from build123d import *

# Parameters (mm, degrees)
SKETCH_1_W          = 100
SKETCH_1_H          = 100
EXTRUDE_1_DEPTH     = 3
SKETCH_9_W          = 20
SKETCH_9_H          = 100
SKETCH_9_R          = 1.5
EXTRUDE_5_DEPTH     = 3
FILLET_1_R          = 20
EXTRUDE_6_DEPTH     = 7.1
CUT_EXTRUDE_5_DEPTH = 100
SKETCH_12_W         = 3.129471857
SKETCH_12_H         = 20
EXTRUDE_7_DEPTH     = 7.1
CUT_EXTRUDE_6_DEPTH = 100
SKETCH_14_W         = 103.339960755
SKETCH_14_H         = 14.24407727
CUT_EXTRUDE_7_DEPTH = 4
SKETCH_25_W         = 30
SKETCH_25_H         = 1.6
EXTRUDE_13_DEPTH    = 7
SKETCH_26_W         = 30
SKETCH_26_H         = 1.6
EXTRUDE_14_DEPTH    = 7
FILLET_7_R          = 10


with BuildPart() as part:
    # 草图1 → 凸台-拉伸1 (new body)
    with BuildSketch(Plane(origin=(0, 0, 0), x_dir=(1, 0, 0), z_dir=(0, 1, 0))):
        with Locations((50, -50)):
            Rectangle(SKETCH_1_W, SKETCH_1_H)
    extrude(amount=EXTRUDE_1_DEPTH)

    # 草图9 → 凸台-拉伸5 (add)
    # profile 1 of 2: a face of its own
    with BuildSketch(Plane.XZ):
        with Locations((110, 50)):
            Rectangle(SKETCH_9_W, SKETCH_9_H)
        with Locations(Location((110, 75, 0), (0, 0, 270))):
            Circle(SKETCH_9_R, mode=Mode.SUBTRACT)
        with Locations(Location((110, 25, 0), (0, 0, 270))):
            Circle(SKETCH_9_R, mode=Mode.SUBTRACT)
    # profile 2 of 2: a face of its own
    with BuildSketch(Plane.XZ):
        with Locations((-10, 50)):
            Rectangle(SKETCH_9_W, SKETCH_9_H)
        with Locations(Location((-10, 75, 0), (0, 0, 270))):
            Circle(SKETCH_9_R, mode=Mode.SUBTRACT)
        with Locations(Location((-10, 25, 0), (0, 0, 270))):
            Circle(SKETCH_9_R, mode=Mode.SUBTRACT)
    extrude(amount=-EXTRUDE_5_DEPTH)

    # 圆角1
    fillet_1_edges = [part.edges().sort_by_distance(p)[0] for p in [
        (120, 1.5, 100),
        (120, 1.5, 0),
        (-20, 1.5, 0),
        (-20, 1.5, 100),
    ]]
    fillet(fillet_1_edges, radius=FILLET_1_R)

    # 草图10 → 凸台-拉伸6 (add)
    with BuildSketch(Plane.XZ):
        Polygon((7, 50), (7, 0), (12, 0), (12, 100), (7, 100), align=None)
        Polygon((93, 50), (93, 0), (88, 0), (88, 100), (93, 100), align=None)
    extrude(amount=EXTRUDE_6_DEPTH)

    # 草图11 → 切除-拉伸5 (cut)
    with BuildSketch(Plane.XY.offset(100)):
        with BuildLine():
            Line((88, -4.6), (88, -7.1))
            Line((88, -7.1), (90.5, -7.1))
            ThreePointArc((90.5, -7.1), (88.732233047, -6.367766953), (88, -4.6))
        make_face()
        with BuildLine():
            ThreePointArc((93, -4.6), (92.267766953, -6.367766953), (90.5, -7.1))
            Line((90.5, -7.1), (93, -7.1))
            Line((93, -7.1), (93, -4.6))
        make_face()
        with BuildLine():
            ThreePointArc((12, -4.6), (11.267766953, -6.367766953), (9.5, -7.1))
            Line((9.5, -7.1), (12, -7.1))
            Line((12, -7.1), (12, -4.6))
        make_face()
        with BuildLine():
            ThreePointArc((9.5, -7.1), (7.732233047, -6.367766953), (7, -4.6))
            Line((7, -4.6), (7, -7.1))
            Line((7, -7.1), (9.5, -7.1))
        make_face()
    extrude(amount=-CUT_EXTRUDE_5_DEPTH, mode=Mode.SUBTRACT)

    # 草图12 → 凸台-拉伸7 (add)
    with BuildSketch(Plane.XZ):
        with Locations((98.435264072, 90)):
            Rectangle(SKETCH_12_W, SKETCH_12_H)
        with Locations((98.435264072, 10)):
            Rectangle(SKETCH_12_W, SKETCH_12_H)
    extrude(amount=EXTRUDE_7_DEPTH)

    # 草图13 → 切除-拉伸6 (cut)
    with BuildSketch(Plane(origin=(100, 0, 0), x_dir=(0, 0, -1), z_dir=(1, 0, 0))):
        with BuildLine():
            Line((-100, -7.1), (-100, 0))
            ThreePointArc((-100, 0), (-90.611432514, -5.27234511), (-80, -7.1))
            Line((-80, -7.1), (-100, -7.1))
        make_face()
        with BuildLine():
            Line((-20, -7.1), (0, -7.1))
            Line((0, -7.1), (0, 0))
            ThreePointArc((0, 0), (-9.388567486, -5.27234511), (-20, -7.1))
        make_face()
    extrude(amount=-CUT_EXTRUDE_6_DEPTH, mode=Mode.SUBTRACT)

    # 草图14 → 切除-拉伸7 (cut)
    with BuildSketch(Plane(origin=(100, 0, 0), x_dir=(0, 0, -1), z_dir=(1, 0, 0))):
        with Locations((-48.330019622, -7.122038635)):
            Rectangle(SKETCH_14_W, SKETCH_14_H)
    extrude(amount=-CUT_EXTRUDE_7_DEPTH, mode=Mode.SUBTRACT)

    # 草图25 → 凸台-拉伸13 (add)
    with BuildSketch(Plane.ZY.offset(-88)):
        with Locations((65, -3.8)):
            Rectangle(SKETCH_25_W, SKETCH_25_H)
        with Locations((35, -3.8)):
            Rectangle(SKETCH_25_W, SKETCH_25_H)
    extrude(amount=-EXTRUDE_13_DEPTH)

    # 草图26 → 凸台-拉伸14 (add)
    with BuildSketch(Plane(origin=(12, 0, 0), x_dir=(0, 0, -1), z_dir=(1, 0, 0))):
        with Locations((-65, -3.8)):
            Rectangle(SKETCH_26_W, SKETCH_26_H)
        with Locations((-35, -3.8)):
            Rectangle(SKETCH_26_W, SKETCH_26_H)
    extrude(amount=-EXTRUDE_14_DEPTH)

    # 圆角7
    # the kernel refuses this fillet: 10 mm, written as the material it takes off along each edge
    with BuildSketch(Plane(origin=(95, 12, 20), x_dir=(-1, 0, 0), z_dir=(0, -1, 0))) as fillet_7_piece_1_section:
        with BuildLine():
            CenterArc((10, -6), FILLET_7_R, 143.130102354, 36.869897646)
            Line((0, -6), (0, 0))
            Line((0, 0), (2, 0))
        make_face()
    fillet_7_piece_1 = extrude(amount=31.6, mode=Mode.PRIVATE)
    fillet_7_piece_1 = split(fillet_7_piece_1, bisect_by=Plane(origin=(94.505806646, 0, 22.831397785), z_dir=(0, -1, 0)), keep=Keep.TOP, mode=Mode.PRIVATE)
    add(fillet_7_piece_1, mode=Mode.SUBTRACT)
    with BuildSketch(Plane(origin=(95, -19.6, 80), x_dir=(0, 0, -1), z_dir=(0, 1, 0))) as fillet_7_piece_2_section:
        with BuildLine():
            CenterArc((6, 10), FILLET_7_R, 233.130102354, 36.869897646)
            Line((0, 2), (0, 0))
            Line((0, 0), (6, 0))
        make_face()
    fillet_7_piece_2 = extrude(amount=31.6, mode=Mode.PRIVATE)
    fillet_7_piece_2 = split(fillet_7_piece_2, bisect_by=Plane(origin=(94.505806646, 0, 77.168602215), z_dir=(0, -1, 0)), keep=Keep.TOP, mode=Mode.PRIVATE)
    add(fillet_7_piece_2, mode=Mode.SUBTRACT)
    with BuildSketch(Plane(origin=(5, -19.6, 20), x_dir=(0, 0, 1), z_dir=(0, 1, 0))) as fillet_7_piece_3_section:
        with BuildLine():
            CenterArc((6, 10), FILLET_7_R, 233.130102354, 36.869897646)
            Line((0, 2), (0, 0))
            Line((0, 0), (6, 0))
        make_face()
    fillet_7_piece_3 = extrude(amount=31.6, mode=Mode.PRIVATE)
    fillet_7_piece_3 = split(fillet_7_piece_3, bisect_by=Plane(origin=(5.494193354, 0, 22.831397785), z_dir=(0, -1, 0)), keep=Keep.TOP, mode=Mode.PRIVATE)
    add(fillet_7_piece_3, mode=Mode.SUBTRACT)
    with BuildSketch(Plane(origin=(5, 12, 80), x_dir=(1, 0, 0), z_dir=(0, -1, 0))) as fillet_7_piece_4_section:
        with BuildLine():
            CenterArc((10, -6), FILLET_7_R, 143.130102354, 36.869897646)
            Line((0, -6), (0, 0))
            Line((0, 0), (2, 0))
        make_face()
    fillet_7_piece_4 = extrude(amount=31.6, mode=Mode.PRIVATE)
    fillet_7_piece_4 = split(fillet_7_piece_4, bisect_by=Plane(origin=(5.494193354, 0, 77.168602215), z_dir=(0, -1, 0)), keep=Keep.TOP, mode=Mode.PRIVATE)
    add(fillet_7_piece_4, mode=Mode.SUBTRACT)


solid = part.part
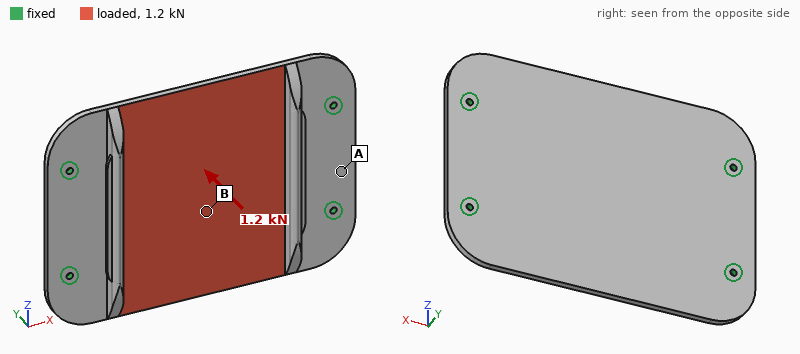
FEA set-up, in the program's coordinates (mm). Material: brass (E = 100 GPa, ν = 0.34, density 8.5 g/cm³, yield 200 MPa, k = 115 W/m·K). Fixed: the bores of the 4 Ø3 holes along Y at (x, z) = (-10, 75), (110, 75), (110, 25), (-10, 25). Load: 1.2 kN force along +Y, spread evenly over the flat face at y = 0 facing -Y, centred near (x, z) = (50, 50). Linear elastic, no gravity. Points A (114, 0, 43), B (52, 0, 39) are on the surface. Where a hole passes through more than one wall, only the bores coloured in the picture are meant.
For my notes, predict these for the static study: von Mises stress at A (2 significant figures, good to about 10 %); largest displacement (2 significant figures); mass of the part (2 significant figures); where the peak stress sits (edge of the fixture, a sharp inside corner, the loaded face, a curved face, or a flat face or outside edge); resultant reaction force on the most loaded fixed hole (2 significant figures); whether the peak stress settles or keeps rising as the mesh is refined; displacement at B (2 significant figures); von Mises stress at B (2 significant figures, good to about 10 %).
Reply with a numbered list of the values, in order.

1. 26 MPa
2. 0.48 mm
3. 400 g
4. edge of the fixture
5. 300 N
6. keeps rising
7. 0.43 mm
8. 62 MPa
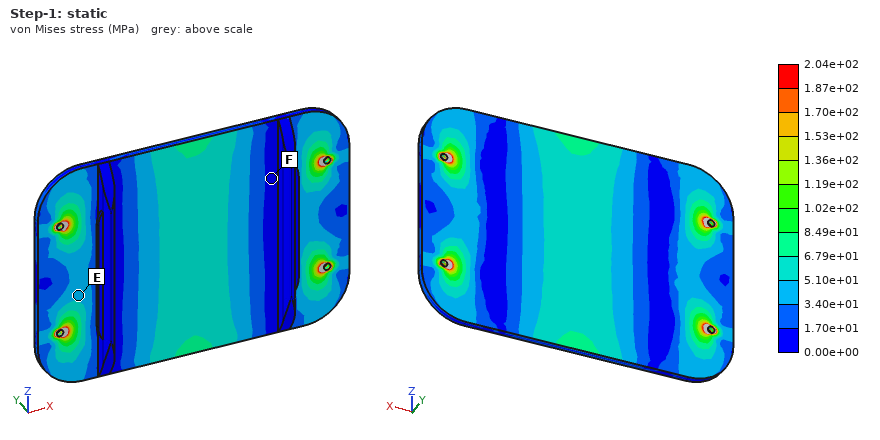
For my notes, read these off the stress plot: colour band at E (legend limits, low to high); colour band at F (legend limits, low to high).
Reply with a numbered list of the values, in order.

1. 3.40e+01 to 5.10e+01 MPa
2. 0.00e+00 to 1.70e+01 MPa
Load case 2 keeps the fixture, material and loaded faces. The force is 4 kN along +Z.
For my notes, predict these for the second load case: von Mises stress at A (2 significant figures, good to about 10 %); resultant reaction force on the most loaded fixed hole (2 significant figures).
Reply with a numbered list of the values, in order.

1. 8.0 MPa
2. 1.1 kN
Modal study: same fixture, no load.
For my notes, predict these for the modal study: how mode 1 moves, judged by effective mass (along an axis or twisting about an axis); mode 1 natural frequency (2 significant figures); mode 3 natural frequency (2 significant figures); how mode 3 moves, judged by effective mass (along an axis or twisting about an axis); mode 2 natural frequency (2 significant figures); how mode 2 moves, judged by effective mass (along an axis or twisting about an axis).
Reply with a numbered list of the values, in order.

1. along Y
2. 620 Hz
3. 1600 Hz
4. twisting about Z
5. 870 Hz
6. twisting about X
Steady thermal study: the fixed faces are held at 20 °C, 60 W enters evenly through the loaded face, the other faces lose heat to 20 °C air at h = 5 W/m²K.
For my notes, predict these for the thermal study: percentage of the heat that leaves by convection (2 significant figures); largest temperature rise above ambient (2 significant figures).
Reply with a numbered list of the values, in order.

1. 5.2 %
2. 45 K
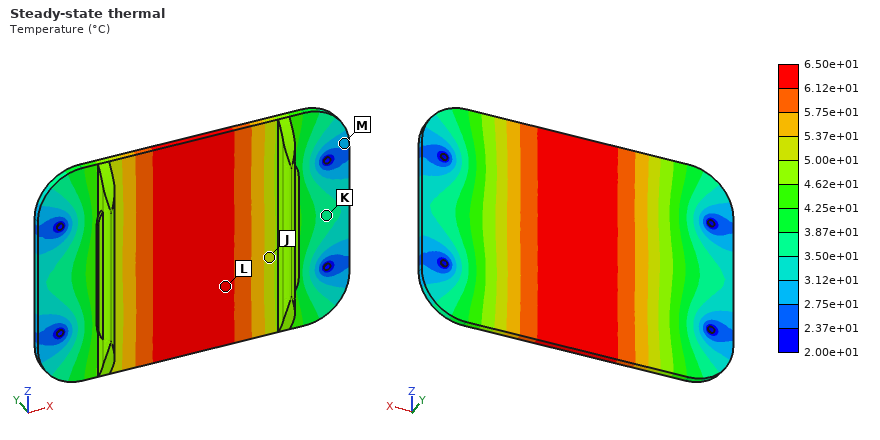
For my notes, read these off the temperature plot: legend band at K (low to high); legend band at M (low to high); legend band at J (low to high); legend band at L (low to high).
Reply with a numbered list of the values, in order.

1. 3.50e+01 to 3.87e+01 °C
2. 2.75e+01 to 3.12e+01 °C
3. 5.00e+01 to 5.37e+01 °C
4. 6.12e+01 to 6.50e+01 °C
